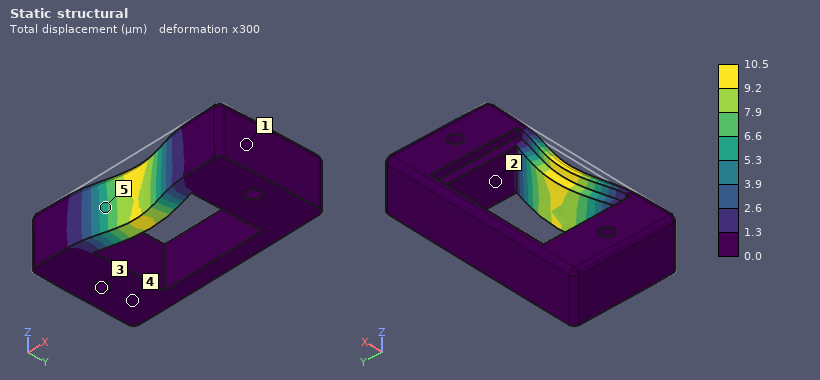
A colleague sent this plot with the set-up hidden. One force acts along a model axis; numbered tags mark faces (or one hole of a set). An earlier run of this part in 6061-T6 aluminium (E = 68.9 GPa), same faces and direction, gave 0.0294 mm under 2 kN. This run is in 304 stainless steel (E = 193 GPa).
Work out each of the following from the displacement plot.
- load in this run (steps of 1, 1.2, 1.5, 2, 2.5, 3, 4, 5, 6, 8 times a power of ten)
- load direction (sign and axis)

2 kN
+Y
